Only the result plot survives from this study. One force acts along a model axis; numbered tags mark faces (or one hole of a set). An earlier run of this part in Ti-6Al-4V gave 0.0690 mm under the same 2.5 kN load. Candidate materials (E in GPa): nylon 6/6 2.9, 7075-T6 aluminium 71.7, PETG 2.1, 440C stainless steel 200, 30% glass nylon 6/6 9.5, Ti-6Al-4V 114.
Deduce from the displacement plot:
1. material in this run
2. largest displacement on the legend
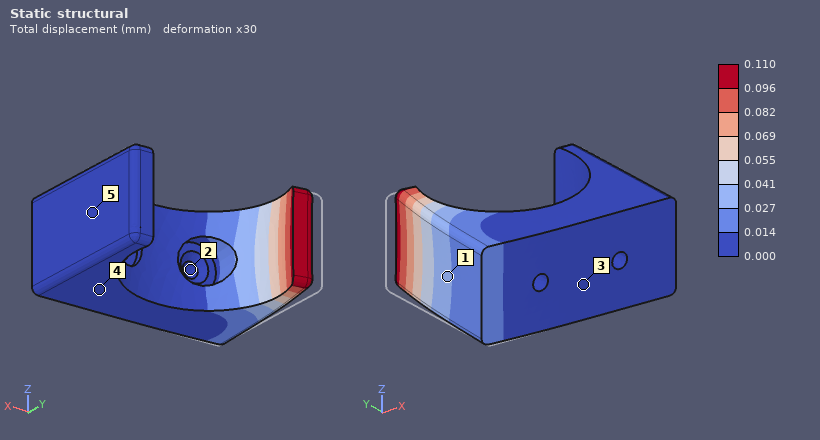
7075-T6 aluminium
0.110 mm
